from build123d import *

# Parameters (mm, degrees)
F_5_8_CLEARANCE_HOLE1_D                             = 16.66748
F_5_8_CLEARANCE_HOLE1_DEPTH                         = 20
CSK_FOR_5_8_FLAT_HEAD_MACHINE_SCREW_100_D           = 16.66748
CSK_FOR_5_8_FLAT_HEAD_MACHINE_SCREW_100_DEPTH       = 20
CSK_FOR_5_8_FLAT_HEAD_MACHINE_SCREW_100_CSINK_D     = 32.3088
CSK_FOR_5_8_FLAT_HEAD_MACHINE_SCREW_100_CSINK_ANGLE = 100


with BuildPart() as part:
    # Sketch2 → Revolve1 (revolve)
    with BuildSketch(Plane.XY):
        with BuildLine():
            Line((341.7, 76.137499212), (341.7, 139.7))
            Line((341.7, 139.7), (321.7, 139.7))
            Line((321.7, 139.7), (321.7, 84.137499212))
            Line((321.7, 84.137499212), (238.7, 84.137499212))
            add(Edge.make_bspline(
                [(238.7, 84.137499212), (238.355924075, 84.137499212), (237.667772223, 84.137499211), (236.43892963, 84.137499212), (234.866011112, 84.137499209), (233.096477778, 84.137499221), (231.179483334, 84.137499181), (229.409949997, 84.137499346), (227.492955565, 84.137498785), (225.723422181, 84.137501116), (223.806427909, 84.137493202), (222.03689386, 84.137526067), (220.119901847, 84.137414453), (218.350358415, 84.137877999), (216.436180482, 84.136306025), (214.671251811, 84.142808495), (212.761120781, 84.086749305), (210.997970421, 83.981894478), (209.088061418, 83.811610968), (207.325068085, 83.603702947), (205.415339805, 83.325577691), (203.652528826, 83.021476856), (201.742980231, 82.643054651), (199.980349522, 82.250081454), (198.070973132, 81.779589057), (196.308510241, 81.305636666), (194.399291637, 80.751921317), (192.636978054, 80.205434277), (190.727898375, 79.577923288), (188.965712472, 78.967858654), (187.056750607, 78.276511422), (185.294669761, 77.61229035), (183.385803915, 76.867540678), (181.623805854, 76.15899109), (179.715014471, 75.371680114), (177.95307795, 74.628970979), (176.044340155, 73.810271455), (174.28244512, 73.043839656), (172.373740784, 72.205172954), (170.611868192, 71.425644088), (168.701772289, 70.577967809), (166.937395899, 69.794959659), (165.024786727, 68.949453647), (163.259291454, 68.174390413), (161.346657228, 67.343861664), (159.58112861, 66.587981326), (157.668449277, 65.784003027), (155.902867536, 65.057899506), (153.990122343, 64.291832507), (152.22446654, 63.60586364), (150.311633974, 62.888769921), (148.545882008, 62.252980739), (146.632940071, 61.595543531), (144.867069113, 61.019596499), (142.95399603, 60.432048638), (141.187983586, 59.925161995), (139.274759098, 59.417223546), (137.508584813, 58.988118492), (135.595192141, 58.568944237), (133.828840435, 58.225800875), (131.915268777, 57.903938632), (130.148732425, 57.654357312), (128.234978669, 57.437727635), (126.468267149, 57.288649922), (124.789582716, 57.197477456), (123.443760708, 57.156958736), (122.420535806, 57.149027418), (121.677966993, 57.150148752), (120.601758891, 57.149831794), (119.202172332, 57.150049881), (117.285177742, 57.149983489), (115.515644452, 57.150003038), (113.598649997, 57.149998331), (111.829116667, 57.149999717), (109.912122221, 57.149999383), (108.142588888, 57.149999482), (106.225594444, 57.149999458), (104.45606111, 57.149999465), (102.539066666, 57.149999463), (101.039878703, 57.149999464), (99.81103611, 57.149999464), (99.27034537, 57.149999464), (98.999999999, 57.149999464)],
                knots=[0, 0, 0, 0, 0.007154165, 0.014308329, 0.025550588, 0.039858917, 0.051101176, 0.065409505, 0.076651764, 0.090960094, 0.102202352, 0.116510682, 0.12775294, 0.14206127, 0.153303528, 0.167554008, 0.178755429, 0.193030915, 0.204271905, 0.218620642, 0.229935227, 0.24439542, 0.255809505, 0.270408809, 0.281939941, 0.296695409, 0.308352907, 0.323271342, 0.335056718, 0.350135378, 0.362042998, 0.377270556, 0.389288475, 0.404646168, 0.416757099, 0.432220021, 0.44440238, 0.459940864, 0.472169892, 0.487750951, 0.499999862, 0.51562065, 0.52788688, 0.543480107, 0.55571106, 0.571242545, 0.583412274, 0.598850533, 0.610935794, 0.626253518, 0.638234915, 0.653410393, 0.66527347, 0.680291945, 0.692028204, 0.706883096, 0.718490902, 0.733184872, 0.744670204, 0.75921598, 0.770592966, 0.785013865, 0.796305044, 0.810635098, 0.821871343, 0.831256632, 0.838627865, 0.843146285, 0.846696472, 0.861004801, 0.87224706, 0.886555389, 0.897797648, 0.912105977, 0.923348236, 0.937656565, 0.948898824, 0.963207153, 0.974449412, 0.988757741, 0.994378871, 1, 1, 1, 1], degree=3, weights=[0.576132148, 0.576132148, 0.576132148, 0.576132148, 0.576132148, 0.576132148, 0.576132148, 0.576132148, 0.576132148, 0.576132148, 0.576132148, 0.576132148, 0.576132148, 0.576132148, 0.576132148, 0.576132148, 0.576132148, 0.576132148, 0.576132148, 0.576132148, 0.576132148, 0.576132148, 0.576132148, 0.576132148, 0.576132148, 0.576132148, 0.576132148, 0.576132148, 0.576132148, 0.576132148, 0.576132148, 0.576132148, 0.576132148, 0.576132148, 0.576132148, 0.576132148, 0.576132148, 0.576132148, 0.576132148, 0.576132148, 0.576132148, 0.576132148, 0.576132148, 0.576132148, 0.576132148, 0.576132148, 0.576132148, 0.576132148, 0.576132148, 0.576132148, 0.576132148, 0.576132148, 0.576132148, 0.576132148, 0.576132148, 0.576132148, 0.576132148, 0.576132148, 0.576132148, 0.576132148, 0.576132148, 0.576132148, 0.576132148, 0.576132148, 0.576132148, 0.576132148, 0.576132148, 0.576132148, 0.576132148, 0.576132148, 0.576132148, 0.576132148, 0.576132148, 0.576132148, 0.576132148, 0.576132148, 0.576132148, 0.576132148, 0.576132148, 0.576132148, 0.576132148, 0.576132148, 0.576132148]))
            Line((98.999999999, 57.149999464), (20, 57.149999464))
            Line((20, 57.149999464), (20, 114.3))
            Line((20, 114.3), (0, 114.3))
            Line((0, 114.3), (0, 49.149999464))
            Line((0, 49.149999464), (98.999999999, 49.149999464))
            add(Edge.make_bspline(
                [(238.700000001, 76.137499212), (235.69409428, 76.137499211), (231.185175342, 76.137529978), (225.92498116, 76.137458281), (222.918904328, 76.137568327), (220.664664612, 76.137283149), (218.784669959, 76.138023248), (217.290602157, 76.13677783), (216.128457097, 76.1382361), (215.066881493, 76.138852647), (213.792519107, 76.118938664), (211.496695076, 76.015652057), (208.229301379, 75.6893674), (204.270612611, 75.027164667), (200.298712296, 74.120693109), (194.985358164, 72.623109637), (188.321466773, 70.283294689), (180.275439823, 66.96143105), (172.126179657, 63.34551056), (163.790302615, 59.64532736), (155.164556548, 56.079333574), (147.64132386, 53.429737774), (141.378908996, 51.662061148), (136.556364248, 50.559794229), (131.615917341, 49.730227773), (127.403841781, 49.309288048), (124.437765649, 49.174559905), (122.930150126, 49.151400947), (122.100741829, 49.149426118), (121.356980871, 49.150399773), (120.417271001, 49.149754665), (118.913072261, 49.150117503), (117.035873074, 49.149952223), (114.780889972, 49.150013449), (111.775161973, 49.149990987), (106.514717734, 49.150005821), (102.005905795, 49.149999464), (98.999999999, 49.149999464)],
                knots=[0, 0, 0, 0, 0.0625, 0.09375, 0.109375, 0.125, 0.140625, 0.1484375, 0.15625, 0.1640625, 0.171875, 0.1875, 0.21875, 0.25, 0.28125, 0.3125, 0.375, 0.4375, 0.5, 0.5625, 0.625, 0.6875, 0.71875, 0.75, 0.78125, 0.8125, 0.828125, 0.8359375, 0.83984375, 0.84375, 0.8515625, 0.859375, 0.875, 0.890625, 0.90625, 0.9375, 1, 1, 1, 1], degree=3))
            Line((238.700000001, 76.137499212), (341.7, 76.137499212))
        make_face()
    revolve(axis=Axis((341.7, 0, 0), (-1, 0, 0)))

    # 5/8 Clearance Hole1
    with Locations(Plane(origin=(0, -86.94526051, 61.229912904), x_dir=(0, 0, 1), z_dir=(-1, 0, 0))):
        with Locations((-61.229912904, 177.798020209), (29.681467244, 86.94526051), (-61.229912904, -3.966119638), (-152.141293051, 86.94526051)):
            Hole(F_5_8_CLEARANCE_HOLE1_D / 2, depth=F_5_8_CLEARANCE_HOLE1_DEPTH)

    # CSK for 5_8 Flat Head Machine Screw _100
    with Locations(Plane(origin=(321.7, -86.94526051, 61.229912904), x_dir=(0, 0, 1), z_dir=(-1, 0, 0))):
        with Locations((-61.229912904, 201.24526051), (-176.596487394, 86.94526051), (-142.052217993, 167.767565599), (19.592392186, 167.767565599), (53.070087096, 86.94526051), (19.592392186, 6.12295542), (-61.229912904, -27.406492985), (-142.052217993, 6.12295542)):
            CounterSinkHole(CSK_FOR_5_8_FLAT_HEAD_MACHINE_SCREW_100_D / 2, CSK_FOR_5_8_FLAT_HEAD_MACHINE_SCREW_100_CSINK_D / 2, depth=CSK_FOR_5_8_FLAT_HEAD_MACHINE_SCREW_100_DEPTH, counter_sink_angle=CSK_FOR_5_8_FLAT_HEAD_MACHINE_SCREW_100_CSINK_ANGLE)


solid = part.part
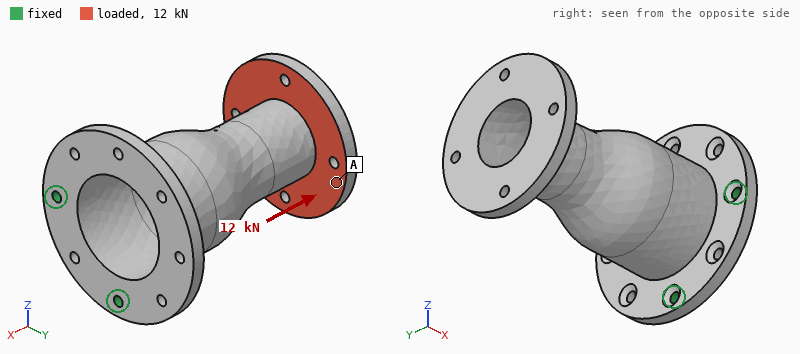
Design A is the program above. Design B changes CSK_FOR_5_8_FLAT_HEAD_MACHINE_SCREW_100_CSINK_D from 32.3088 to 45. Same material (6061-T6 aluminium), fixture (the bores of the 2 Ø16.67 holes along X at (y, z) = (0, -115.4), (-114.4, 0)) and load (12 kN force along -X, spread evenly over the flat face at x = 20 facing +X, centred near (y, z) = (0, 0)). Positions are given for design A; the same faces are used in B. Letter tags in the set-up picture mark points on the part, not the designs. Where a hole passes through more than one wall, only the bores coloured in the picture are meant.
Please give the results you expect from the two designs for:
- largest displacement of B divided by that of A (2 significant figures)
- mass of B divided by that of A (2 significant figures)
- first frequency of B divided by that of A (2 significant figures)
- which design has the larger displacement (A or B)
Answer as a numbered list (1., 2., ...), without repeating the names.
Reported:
1. 1.6
2. 0.98
3. 0.80
4. B
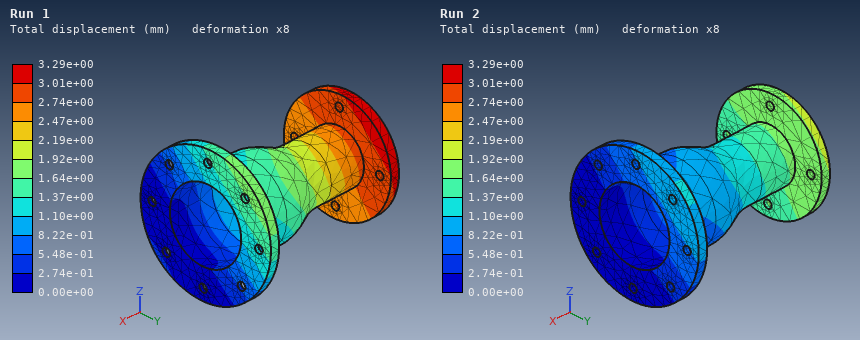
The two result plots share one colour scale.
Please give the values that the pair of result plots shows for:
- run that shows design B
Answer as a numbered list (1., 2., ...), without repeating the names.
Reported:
1. Run 1
